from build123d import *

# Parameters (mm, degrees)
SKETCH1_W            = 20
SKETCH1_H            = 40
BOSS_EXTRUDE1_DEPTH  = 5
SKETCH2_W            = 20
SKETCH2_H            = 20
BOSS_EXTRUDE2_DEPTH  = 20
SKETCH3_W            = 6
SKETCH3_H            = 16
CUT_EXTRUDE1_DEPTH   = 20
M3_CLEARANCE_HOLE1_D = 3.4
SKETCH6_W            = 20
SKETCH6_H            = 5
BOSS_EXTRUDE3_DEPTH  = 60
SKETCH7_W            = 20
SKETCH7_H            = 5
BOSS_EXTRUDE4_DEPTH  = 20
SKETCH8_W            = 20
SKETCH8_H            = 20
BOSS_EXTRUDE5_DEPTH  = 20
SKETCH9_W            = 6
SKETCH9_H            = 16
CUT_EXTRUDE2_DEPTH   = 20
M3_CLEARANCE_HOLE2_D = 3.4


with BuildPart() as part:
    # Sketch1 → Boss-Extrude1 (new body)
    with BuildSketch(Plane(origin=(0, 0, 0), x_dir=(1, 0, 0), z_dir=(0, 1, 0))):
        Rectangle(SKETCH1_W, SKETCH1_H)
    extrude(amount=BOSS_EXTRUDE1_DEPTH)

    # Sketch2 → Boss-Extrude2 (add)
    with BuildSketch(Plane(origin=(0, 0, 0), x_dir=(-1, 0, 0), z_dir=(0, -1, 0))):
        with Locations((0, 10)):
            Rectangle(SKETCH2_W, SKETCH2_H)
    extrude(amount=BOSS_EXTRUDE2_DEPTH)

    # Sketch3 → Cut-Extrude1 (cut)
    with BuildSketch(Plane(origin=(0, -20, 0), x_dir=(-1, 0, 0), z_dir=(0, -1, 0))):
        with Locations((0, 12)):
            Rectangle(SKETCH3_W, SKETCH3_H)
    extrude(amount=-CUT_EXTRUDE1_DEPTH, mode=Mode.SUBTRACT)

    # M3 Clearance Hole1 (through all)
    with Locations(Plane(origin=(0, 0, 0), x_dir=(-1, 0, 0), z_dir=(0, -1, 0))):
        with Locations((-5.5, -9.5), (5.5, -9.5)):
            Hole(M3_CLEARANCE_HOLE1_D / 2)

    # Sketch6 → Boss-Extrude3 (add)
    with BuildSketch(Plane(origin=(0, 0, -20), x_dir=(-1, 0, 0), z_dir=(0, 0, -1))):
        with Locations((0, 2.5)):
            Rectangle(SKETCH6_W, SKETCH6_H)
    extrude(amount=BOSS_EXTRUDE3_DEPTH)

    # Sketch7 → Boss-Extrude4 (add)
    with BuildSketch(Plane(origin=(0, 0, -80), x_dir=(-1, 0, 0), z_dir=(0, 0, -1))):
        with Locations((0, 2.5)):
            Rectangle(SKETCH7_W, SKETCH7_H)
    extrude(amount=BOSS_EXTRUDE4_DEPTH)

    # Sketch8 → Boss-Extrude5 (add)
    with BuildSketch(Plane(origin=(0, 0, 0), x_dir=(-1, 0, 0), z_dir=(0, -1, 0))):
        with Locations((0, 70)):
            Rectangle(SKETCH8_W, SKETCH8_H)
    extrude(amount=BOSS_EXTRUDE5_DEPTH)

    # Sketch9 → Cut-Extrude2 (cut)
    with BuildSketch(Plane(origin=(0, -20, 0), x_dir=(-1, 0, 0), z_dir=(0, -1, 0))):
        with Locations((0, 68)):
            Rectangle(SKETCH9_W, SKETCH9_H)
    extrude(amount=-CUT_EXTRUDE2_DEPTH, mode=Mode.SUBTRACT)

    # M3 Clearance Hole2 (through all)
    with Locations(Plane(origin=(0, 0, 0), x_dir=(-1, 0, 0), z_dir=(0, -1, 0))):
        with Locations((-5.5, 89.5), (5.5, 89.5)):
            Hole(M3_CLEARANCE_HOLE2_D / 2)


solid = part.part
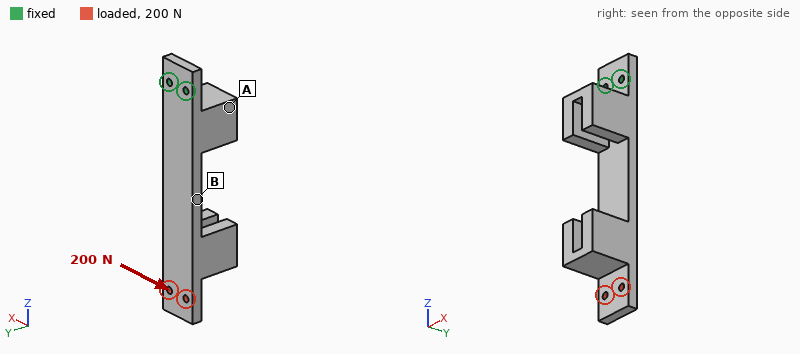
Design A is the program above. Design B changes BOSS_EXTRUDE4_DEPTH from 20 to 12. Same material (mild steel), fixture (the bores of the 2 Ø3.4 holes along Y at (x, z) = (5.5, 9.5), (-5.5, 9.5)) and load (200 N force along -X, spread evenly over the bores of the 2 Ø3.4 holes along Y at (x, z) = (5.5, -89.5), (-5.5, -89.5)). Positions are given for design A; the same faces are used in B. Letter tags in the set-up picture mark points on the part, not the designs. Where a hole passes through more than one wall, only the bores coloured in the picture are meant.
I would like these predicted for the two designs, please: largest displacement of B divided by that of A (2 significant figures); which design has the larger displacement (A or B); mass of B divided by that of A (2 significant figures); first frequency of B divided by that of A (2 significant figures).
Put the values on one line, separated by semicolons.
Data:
0.90; A; 0.97; 1.1
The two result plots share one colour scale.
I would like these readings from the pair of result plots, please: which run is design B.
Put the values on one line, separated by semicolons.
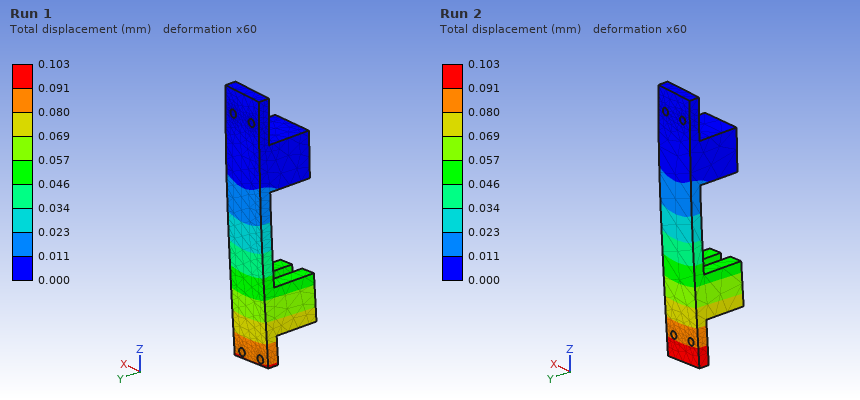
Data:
Run 1
